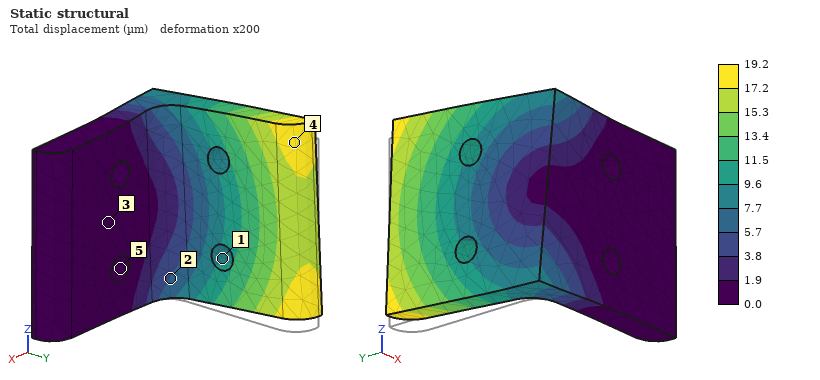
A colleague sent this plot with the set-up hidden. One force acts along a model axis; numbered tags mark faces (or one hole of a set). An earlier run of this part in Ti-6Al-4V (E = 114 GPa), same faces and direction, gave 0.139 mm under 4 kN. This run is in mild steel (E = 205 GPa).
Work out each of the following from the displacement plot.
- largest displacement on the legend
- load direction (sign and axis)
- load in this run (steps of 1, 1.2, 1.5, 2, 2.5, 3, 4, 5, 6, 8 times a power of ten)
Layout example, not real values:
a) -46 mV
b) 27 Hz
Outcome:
a) 19.2 µm
b) +Z
c) 1 kN
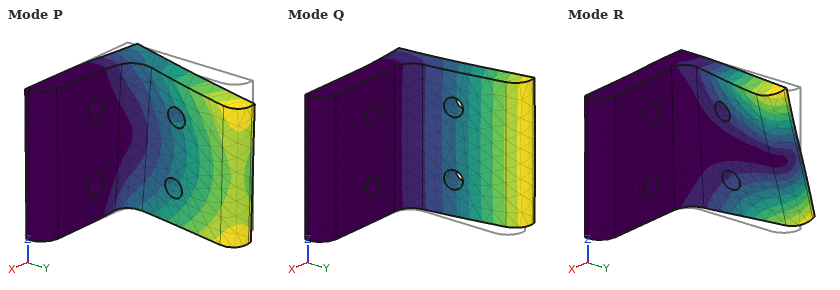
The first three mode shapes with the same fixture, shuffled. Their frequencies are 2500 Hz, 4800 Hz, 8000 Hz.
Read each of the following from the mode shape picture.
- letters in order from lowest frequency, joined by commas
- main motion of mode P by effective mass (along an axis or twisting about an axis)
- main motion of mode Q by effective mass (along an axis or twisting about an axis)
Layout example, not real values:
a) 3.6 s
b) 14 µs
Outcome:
a) Q, P, R
b) along Z
c) along X
